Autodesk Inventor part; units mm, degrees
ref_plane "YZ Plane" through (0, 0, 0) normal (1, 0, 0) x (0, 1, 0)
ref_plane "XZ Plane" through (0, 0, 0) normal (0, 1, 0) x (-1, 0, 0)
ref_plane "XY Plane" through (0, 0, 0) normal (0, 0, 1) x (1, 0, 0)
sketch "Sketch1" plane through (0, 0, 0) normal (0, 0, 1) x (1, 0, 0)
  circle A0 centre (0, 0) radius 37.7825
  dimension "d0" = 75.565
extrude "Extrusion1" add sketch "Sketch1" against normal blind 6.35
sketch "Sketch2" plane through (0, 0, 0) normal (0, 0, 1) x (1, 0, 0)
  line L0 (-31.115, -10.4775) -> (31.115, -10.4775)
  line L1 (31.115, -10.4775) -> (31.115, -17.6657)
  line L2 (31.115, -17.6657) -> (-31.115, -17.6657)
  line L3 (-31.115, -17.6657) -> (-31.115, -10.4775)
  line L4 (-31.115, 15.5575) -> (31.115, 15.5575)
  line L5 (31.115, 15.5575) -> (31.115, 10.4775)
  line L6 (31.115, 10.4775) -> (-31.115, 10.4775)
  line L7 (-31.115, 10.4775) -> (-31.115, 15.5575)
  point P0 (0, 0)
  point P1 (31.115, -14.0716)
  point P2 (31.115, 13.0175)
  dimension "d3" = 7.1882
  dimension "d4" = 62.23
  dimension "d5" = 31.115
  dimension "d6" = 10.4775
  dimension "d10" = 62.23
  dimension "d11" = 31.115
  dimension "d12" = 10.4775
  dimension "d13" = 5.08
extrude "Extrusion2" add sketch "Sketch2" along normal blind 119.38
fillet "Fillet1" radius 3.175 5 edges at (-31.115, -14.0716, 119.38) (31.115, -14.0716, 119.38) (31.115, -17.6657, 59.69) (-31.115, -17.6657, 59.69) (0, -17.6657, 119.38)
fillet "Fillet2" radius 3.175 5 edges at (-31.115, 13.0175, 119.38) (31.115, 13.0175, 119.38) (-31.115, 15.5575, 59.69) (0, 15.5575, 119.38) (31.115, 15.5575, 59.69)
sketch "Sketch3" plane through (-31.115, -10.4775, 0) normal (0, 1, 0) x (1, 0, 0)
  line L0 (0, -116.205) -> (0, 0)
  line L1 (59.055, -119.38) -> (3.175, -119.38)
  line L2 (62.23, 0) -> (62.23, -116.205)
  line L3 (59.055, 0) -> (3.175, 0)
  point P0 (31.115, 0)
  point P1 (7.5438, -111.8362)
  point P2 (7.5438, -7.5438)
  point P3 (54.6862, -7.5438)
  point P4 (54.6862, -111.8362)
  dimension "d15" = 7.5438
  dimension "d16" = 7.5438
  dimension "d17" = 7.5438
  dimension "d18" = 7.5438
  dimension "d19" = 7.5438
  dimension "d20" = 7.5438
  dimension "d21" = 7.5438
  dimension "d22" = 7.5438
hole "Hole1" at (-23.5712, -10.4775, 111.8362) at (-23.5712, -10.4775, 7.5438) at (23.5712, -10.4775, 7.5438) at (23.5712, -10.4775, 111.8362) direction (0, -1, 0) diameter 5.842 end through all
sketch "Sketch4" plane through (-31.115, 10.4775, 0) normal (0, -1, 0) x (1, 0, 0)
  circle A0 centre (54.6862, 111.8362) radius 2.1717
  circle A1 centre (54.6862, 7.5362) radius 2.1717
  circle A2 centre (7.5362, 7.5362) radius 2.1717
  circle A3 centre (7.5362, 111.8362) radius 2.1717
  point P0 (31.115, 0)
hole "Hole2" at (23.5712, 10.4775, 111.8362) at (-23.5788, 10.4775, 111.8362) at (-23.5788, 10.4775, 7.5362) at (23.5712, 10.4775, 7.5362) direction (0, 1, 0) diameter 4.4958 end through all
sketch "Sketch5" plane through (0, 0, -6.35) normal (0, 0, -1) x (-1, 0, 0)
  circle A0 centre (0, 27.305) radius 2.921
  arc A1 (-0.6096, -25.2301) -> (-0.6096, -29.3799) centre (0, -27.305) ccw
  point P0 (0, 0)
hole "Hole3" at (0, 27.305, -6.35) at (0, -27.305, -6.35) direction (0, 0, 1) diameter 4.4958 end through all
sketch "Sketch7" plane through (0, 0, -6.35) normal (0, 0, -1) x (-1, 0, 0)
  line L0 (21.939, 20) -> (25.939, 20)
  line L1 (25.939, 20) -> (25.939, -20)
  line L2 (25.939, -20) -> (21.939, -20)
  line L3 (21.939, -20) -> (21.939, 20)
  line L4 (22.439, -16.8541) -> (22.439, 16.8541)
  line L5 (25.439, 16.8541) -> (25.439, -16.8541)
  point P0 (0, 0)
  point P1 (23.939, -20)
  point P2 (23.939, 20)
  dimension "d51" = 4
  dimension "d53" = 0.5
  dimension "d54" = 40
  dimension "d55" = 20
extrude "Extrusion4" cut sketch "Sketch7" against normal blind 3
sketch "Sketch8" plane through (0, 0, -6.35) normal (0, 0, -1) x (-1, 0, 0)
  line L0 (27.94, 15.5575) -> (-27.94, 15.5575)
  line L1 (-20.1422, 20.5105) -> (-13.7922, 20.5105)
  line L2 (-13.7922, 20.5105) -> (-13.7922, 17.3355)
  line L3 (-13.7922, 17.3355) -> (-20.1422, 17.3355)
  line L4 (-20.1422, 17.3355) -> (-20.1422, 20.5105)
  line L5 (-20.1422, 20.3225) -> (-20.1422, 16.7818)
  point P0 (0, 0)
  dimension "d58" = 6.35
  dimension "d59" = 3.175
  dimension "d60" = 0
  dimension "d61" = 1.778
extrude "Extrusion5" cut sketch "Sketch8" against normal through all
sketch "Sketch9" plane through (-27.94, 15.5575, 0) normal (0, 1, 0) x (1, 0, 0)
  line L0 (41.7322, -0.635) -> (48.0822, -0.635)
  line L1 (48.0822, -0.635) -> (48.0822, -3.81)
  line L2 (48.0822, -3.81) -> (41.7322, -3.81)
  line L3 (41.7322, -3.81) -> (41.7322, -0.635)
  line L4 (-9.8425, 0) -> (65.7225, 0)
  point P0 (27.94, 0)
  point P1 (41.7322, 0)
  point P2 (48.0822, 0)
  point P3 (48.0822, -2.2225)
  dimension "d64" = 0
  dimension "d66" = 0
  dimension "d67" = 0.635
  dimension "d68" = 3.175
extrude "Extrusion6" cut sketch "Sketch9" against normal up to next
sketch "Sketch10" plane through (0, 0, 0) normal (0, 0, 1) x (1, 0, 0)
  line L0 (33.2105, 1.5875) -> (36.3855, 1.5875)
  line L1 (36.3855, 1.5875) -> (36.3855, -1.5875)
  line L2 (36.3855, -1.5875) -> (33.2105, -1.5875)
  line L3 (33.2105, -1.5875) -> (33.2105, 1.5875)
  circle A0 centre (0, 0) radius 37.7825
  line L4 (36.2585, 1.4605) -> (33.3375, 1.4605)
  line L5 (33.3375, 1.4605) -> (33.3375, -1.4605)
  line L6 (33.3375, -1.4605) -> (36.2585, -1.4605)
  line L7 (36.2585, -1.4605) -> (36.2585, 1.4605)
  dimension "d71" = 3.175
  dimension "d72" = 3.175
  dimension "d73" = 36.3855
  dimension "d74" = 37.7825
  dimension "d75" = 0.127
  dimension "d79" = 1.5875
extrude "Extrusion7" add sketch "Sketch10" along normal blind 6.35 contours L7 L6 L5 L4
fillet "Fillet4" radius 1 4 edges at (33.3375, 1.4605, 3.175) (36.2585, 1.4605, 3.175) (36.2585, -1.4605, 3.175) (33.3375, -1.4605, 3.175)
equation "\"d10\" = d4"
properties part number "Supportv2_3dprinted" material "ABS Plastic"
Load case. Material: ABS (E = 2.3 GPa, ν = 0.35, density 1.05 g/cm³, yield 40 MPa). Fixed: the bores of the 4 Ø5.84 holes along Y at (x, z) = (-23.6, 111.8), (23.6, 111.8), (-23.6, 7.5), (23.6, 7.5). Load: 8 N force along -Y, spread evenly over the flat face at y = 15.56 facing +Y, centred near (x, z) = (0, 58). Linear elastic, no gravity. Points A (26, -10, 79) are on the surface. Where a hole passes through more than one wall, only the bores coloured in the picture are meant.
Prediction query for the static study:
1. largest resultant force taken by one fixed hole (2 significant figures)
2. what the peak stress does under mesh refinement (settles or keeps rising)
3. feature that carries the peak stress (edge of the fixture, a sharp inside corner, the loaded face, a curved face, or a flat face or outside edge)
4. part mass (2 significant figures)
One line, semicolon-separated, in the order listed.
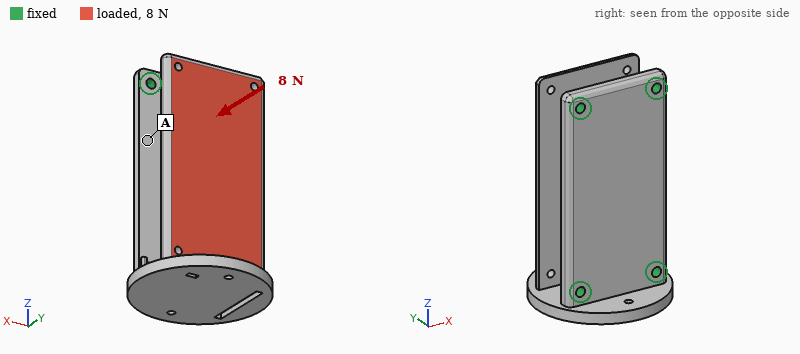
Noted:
4.3 N; keeps rising; a sharp inside corner; 120 g
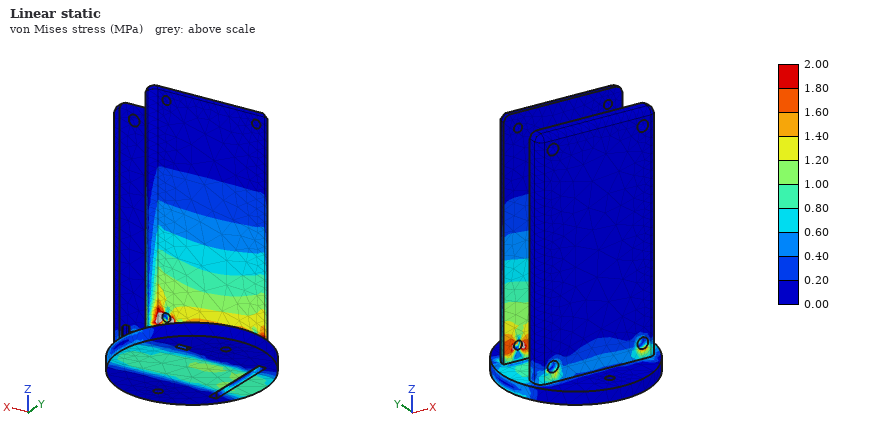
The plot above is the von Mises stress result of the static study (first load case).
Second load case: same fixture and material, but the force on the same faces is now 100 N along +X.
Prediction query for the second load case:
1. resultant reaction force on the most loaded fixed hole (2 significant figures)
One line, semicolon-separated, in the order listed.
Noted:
130 N
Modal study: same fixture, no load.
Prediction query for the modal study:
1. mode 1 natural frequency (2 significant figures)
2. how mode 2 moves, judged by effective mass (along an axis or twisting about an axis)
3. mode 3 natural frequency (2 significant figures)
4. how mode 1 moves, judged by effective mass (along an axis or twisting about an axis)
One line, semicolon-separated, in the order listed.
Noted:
69 Hz; along X; 340 Hz; along Y
